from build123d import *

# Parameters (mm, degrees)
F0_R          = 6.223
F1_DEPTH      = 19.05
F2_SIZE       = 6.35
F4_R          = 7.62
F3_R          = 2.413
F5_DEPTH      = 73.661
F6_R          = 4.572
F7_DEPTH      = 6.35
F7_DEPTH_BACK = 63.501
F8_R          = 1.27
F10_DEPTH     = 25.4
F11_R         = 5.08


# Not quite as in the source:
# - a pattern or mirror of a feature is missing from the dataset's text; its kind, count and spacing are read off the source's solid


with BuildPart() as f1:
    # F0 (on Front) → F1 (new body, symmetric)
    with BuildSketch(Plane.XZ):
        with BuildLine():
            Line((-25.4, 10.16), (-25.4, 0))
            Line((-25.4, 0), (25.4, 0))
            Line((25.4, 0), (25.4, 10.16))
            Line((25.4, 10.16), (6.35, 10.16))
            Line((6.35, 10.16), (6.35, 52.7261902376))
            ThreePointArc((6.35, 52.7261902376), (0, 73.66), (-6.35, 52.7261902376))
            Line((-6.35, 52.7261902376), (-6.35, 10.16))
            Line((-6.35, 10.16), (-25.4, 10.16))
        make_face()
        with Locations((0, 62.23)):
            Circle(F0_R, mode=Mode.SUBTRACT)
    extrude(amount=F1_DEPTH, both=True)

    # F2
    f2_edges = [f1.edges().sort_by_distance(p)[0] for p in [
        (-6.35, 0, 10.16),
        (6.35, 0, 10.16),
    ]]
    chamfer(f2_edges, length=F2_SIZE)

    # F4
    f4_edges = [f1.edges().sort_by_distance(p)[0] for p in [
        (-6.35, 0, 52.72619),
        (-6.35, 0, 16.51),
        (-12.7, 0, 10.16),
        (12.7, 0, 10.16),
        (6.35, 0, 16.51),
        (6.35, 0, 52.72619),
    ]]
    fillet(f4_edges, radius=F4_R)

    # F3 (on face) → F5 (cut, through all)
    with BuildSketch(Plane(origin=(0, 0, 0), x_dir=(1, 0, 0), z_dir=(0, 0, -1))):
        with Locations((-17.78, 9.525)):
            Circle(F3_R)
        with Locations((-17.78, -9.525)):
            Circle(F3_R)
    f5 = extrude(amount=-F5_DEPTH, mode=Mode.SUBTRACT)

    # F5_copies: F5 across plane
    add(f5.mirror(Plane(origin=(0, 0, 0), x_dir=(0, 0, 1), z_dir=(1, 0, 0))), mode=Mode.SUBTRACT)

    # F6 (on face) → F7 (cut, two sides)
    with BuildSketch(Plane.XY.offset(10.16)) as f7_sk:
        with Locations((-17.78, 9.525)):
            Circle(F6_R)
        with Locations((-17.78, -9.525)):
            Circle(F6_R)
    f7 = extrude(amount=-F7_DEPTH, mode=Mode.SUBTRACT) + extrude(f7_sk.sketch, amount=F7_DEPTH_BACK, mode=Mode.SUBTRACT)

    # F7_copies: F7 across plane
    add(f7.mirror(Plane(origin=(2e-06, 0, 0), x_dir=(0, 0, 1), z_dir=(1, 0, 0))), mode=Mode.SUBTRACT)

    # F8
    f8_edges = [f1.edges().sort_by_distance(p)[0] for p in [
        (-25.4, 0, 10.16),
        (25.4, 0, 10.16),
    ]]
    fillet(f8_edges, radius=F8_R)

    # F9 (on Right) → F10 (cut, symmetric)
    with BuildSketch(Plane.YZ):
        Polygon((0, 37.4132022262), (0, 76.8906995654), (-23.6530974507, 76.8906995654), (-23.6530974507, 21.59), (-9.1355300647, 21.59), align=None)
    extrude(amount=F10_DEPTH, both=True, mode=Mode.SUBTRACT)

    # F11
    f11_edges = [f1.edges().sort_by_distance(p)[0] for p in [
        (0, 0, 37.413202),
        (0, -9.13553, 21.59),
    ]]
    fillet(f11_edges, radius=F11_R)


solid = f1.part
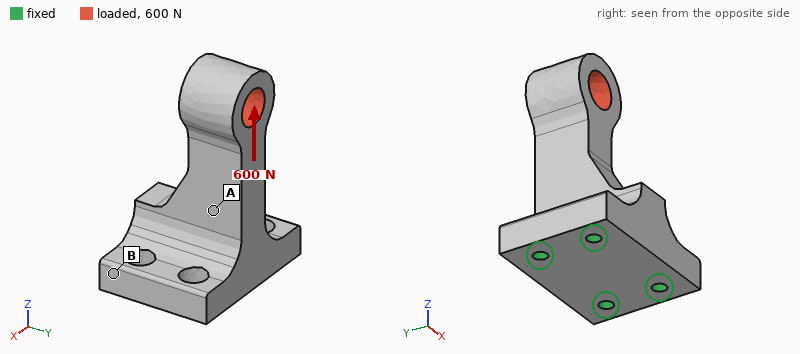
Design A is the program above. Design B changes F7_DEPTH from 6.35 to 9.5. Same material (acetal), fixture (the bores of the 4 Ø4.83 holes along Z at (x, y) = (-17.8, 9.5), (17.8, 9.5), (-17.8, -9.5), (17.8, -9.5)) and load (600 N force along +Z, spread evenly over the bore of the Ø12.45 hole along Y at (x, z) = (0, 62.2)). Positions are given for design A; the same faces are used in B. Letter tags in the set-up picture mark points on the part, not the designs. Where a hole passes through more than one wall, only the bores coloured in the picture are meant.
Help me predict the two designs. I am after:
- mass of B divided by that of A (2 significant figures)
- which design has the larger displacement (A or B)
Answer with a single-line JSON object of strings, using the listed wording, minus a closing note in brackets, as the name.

{"mass of B divided by that of A": "0.98", "which design has the larger displacement": "B"}
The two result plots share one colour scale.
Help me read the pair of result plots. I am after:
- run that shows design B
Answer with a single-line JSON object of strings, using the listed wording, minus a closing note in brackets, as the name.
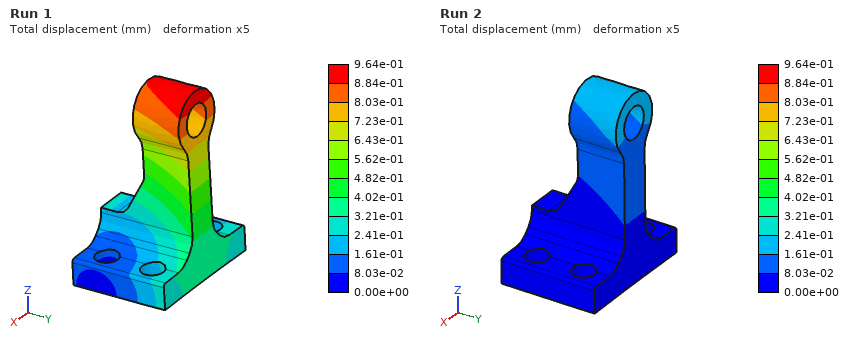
{"run that shows design B": "Run 1"}
